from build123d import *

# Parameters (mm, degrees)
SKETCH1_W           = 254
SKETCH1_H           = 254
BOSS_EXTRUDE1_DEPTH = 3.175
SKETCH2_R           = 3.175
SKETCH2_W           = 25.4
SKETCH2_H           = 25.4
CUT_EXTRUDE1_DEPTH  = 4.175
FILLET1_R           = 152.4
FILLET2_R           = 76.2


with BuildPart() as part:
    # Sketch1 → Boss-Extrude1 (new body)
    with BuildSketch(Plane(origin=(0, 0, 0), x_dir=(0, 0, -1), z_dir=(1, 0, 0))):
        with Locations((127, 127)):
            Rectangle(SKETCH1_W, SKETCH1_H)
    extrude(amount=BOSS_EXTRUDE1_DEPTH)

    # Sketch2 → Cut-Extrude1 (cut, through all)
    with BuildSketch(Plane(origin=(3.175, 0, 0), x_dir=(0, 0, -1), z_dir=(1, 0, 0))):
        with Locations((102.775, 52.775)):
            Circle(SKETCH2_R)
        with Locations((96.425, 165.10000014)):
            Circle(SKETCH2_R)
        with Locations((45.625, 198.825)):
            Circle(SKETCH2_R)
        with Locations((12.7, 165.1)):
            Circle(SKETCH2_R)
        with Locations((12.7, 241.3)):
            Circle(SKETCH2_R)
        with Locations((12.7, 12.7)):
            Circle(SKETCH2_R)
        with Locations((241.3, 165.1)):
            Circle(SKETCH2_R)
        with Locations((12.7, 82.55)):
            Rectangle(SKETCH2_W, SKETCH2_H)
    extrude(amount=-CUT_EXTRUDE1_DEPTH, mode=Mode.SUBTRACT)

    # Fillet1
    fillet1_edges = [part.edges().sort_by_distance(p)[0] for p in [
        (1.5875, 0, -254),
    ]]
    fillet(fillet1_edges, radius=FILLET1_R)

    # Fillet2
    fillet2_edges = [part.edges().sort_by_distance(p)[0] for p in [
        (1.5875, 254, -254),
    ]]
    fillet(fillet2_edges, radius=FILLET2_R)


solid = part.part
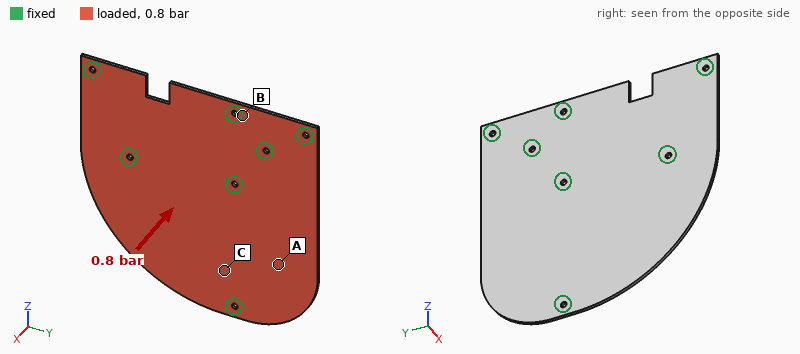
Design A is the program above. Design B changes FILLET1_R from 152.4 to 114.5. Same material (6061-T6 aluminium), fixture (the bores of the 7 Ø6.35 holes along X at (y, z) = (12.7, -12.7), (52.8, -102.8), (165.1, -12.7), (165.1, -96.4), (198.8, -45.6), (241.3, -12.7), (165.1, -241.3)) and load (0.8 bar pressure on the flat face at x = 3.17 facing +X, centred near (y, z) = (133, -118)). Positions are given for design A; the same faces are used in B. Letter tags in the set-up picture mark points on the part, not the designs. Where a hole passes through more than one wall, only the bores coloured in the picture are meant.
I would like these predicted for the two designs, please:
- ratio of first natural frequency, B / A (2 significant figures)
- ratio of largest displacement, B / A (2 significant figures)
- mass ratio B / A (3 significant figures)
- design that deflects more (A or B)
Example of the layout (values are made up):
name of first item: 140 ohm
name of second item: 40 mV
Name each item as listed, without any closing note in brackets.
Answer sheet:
ratio of first natural frequency, B / A: 0.86
ratio of largest displacement, B / A: 1.5
mass ratio B / A: 1.04
design that deflects more: B
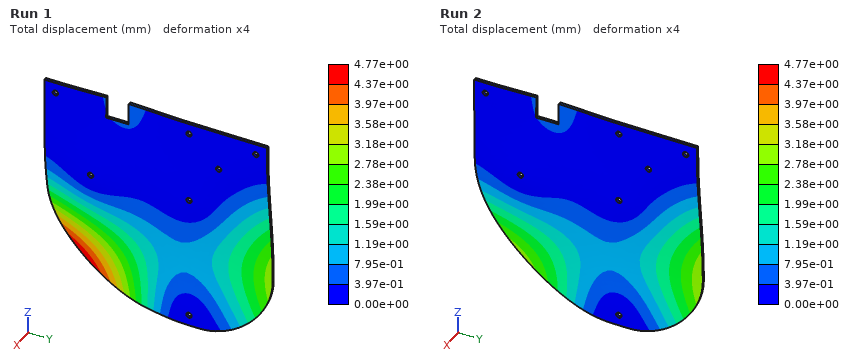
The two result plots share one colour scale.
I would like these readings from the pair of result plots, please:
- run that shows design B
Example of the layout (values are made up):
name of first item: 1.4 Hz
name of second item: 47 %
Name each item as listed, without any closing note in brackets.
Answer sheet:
run that shows design B: Run 1
